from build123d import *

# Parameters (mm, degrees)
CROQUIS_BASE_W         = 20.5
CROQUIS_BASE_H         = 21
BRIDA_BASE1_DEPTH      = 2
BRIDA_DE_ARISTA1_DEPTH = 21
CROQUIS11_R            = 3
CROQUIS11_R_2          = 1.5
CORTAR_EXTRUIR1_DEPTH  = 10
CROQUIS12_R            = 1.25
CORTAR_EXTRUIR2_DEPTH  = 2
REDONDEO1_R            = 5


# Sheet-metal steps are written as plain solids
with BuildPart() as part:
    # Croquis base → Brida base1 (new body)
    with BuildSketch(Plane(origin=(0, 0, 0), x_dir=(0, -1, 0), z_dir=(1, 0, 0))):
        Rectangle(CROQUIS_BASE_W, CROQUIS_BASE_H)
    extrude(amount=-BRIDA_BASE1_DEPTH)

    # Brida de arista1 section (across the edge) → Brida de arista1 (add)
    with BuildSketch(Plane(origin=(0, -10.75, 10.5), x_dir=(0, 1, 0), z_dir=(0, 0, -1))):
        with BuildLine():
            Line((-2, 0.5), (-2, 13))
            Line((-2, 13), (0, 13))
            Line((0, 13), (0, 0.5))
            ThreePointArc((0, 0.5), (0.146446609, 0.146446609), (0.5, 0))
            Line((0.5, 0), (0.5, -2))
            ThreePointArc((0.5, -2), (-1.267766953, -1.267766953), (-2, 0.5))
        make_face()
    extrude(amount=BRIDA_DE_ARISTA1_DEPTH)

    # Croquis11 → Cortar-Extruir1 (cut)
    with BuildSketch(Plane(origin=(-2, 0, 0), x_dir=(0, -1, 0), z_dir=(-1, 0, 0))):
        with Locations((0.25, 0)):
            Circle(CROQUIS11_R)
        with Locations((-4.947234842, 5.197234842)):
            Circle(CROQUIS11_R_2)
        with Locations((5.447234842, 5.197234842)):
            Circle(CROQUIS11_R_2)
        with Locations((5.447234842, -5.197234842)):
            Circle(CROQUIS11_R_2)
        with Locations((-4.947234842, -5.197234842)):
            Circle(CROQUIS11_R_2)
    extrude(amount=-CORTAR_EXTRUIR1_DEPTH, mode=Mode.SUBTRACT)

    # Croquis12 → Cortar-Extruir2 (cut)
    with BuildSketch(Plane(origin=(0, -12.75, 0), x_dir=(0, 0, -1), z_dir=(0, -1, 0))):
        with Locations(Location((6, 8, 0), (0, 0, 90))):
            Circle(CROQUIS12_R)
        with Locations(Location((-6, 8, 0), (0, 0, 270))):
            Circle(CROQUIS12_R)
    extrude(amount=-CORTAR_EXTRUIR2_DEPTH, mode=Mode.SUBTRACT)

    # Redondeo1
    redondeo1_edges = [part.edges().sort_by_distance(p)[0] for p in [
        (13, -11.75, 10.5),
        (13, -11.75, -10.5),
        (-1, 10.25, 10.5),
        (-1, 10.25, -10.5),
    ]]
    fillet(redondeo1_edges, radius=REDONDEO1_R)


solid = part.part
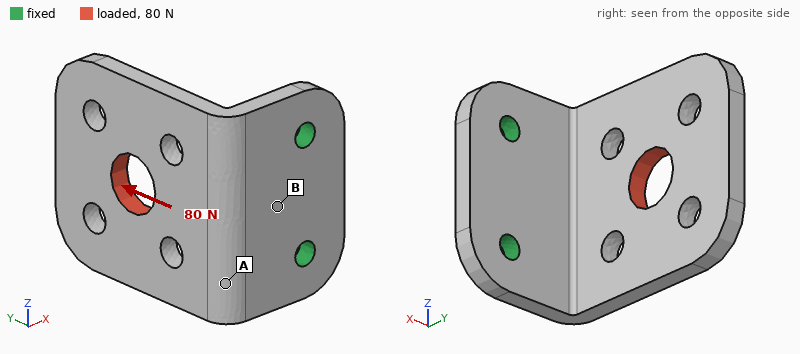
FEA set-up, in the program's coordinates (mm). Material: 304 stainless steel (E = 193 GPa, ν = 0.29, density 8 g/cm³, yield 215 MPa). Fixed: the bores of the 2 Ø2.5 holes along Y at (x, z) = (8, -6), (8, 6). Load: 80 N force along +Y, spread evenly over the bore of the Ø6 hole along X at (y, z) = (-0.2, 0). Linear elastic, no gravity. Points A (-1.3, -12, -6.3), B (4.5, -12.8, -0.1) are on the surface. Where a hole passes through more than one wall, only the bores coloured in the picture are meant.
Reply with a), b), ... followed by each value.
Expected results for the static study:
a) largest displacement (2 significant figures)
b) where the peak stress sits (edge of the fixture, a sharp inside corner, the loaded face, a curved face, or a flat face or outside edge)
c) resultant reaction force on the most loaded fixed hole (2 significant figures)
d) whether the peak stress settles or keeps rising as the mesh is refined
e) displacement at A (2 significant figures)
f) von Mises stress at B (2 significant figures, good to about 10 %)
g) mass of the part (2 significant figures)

a) 26 µm
b) edge of the fixture
c) 40 N
d) keeps rising
e) 7.0 µm
f) 24 MPa
g) 10 g
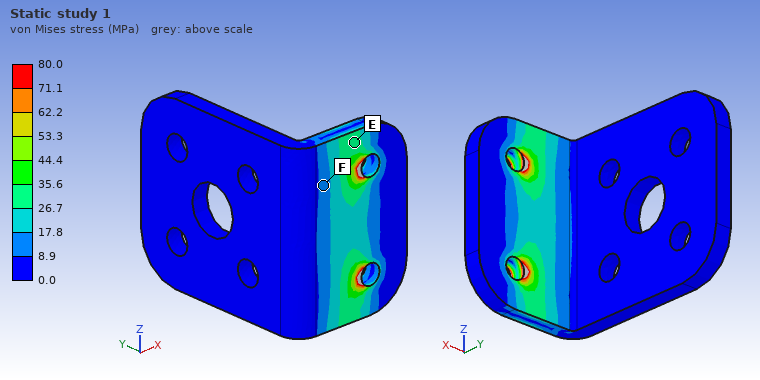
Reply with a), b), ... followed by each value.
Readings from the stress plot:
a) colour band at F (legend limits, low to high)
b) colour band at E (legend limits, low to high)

a) 8.9 to 17.8 MPa
b) 26.7 to 35.6 MPa
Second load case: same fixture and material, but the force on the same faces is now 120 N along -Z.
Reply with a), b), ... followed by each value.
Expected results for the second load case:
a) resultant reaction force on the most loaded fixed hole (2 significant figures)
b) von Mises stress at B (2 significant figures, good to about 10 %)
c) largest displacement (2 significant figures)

a) 140 N
b) 24 MPa
c) 27 µm
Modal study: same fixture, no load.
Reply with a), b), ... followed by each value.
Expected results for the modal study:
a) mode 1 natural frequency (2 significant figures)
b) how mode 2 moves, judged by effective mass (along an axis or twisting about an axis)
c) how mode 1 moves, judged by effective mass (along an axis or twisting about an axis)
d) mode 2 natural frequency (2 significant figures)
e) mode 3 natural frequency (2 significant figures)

a) 2200 Hz
b) along Z
c) along X
d) 4800 Hz
e) 7900 Hz
